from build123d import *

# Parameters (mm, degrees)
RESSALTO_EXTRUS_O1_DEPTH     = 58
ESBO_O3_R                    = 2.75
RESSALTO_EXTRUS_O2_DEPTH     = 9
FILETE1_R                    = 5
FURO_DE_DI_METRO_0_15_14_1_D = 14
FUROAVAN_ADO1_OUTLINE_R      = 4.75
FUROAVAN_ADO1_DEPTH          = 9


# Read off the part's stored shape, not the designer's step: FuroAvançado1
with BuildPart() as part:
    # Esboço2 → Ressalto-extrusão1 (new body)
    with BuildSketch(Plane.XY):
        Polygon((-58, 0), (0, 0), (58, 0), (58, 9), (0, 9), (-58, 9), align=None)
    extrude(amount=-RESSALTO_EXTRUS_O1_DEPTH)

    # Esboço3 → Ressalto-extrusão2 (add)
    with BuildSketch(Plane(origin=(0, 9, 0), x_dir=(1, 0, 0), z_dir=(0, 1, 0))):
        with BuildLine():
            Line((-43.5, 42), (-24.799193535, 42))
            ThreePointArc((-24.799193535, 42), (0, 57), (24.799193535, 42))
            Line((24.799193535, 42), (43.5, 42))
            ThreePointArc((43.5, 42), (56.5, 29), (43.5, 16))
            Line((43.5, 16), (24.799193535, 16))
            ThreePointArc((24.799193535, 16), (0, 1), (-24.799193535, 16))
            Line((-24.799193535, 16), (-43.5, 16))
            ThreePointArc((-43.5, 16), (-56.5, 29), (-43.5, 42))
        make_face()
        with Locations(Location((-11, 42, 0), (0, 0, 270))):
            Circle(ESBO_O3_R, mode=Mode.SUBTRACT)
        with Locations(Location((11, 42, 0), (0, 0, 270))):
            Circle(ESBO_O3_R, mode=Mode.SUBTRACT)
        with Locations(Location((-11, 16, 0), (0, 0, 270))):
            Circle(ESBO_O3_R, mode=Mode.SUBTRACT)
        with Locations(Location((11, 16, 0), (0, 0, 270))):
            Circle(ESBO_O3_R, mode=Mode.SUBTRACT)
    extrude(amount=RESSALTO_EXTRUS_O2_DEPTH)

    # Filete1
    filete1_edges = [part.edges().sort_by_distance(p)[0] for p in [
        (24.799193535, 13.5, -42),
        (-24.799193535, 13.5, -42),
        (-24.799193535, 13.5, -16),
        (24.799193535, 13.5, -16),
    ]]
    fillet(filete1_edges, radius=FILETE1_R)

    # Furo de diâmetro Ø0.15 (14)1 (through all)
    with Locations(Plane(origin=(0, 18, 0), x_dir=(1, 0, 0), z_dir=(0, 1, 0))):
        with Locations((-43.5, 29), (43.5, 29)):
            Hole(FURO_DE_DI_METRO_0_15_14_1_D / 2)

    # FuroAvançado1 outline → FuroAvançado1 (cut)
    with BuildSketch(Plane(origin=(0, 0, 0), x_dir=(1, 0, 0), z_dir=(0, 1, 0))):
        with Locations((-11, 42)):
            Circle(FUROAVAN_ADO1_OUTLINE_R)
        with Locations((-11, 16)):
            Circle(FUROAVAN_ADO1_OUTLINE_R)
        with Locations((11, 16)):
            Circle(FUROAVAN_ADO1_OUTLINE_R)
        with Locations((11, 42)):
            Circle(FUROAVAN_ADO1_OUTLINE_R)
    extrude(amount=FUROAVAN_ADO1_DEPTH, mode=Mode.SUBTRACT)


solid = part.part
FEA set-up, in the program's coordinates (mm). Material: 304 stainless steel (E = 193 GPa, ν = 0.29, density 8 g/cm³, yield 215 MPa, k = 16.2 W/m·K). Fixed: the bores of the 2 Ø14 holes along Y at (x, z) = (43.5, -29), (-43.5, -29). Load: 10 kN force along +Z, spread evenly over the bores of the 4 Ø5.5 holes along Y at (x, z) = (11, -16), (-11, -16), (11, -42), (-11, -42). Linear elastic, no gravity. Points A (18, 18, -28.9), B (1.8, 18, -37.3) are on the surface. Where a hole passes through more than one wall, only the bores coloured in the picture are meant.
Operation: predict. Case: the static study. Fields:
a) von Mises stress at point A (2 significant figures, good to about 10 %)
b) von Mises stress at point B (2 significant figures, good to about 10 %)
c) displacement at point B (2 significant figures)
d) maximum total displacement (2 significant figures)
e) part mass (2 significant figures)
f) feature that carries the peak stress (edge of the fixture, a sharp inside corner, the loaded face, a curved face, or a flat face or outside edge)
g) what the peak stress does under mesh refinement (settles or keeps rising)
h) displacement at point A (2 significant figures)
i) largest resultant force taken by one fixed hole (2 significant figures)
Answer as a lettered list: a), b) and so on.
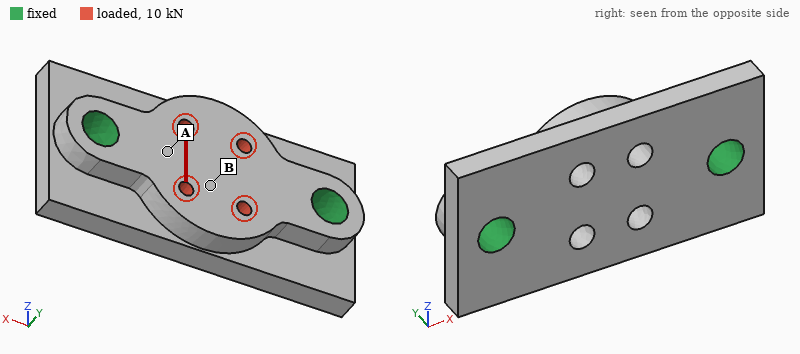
a) 21 MPa
b) 6.2 MPa
c) 6.5 µm
d) 8.4 µm
e) 690 g
f) edge of the fixture
g) keeps rising
h) 4.9 µm
i) 5.0 kN
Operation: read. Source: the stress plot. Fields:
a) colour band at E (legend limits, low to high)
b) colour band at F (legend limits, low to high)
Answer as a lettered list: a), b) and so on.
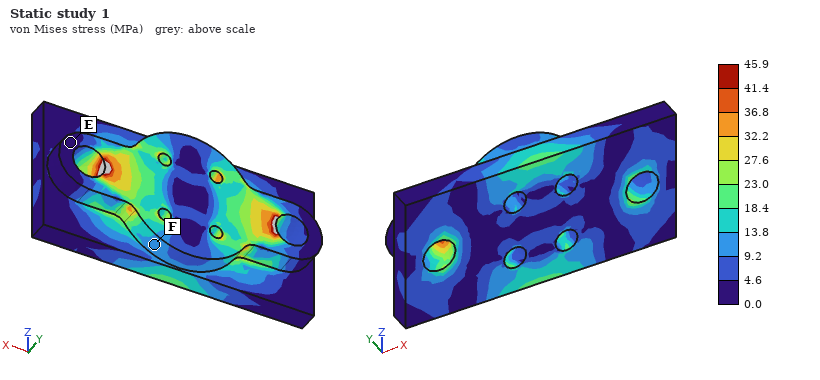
a) 0.0 to 4.6 MPa
b) 9.2 to 13.8 MPa
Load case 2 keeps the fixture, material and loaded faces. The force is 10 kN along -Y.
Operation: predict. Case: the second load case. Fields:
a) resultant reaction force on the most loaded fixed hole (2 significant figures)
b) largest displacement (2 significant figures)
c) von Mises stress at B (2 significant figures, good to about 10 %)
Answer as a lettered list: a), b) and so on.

a) 5.0 kN
b) 11 µm
c) 19 MPa
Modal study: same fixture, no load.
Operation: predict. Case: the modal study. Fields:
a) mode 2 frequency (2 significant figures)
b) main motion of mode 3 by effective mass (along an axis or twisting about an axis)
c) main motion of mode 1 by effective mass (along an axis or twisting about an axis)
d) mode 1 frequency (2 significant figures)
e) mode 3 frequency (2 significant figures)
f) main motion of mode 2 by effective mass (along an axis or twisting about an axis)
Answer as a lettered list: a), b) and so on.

a) 8800 Hz
b) along Z
c) twisting about X
d) 8300 Hz
e) 13 kHz
f) along Y
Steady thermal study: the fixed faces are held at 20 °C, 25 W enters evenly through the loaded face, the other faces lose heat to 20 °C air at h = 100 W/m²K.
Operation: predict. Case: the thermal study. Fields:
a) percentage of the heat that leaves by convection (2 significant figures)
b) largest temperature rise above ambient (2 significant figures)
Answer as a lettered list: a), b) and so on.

a) 58 %
b) 25 K
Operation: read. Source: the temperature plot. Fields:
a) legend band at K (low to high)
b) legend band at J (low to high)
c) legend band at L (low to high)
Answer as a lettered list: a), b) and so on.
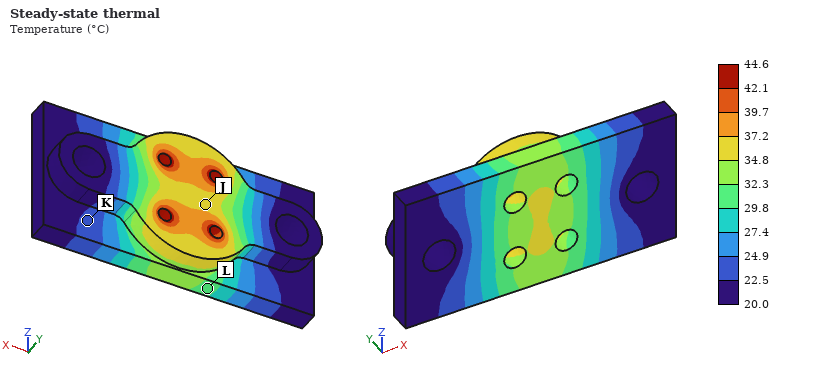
a) 22.5 to 24.9 °C
b) 34.8 to 37.2 °C
c) 29.8 to 32.3 °C
